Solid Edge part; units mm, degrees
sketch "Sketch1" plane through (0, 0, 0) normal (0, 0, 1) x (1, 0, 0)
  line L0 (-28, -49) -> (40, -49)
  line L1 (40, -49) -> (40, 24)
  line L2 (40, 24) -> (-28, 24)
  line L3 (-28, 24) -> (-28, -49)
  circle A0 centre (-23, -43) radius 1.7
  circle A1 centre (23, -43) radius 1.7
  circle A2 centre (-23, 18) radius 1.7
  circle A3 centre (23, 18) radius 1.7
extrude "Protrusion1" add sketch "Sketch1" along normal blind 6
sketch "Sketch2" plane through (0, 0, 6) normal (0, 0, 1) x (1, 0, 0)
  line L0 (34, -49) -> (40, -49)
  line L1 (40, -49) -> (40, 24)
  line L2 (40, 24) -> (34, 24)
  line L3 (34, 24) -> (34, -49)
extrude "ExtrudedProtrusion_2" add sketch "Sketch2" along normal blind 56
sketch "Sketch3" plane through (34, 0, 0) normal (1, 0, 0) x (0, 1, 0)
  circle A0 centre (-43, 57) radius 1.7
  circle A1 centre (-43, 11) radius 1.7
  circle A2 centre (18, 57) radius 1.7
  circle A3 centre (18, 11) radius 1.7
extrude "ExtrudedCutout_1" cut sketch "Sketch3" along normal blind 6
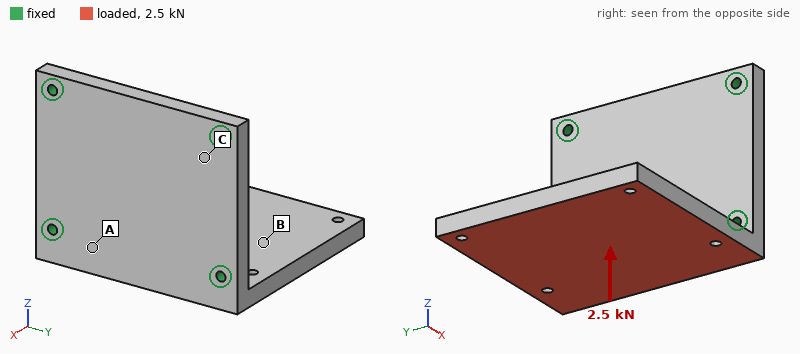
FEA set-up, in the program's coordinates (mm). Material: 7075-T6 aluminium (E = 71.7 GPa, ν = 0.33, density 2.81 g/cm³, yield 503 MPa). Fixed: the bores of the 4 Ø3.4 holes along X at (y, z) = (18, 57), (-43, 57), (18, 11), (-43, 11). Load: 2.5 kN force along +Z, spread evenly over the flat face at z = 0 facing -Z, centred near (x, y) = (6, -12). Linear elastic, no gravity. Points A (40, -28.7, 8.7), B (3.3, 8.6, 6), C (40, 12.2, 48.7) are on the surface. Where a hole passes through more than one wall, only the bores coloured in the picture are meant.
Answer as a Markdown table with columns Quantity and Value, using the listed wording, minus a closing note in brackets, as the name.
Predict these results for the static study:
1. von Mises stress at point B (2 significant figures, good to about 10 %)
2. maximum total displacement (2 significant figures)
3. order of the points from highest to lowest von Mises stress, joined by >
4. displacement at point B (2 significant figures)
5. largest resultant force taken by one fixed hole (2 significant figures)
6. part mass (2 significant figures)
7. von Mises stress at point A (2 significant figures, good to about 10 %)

| Quantity | Value |
|---|---|
| von Mises stress at point B | 40 MPa |
| maximum total displacement | 1.4 mm |
| order of the points from highest to lowest von Mises stress, joined by > | A > B > C |
| displacement at point B | 0.58 mm |
| largest resultant force taken by one fixed hole | 890 N |
| part mass | 150 g |
| von Mises stress at point A | 120 MPa |
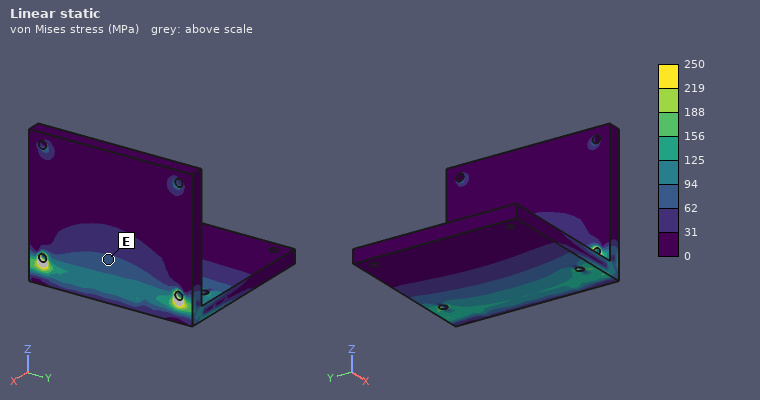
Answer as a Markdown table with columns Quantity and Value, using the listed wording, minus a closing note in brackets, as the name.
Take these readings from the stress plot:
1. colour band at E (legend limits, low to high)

| Quantity | Value |
|---|---|
| colour band at E | 62 to 94 MPa |
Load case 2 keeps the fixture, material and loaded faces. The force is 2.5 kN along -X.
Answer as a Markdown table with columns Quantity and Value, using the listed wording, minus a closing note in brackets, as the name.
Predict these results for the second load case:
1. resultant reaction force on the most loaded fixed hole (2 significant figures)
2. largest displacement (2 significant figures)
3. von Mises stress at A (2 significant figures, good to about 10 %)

| Quantity | Value |
|---|---|
| resultant reaction force on the most loaded fixed hole | 1.4 kN |
| largest displacement | 0.26 mm |
| von Mises stress at A | 24 MPa |
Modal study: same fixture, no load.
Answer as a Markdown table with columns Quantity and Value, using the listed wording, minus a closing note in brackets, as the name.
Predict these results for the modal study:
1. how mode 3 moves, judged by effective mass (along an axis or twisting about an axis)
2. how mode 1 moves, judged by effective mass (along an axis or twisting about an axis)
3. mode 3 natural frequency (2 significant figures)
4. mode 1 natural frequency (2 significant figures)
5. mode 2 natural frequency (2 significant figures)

| Quantity | Value |
|---|---|
| how mode 3 moves, judged by effective mass | along Y |
| how mode 1 moves, judged by effective mass | along Z |
| mode 3 natural frequency | 5000 Hz |
| mode 1 natural frequency | 930 Hz |
| mode 2 natural frequency | 2400 Hz |
